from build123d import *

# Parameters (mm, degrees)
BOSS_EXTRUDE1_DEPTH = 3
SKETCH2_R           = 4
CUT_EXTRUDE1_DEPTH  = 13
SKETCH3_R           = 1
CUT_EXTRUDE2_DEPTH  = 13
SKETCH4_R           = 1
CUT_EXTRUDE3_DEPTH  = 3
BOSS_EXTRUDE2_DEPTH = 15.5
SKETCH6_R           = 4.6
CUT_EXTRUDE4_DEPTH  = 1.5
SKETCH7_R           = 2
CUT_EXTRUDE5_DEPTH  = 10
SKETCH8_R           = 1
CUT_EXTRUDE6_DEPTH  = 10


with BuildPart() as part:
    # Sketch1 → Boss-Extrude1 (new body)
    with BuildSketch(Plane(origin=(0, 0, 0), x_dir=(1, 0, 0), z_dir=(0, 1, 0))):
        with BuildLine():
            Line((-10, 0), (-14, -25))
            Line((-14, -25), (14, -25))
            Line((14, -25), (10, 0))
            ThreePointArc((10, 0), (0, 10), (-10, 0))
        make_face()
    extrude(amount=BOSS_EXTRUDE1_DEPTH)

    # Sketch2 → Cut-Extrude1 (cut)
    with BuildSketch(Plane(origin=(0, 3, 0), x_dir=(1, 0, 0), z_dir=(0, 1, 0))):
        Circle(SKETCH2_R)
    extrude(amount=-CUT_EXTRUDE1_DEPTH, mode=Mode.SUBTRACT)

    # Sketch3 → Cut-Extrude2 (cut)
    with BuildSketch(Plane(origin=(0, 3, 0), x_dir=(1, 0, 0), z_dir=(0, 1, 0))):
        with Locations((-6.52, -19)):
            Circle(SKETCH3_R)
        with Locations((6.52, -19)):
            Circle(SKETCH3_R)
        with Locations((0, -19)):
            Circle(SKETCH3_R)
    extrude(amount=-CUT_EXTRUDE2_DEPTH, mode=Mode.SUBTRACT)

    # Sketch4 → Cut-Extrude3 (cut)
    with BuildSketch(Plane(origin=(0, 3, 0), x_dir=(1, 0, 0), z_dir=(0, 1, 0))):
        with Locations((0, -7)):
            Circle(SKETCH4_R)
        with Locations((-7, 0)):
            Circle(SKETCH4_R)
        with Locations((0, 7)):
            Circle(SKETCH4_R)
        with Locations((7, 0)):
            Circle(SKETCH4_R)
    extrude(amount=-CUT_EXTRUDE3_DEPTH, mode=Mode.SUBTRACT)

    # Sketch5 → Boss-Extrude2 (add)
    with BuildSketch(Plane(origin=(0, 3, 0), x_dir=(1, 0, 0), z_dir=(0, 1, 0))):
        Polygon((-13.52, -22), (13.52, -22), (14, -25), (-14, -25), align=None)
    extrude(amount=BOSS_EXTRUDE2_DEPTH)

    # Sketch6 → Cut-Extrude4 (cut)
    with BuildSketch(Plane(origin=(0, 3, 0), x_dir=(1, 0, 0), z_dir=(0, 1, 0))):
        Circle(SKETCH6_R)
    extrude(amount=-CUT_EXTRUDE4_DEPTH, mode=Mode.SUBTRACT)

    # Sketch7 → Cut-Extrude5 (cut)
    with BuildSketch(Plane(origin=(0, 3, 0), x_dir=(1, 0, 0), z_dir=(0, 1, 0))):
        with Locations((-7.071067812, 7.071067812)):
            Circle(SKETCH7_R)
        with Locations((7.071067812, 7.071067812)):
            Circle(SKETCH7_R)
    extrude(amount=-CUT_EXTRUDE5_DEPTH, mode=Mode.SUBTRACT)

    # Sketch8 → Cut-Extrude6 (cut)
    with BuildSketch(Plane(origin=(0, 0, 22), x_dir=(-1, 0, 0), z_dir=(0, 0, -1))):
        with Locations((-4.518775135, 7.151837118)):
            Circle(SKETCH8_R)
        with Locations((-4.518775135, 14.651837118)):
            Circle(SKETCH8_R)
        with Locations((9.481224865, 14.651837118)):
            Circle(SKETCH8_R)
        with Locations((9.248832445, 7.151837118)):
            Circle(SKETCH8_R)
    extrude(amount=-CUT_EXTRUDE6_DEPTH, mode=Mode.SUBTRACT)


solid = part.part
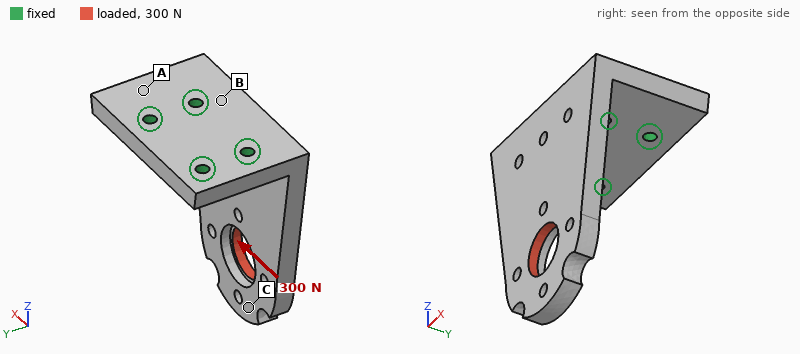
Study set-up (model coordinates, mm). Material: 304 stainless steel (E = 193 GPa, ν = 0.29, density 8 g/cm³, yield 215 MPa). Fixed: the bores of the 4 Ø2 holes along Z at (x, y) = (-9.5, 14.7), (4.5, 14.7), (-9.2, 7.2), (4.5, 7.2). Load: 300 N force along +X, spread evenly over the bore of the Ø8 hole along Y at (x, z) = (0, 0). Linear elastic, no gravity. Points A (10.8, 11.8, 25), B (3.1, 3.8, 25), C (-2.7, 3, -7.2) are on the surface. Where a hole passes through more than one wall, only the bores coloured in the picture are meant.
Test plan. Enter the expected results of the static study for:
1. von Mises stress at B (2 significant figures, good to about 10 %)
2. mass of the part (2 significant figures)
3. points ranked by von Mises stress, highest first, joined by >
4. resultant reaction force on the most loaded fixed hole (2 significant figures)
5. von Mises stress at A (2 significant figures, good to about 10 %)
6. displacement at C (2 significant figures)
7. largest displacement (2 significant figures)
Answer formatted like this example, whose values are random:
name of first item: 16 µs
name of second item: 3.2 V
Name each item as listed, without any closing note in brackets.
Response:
von Mises stress at B: 35 MPa
mass of the part: 26 g
points ranked by von Mises stress, highest first, joined by >: B > A > C
resultant reaction force on the most loaded fixed hole: 500 N
von Mises stress at A: 24 MPa
displacement at C: 23 µm
largest displacement: 25 µm
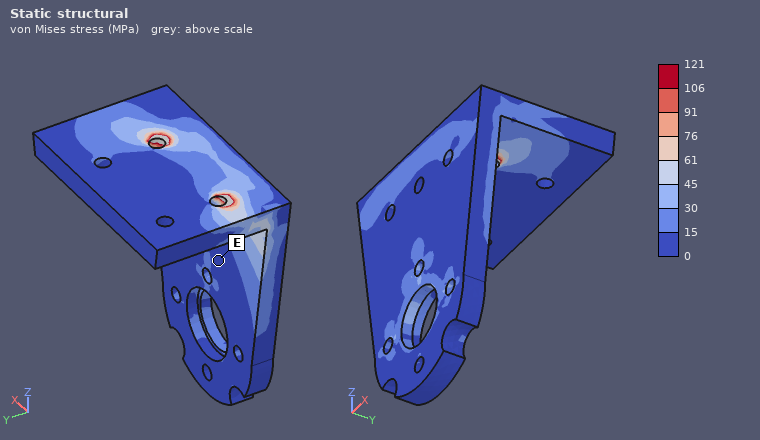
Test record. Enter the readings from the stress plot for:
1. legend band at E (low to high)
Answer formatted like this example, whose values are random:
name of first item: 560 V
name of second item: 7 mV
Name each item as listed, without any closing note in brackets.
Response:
legend band at E: 0 to 15 MPa
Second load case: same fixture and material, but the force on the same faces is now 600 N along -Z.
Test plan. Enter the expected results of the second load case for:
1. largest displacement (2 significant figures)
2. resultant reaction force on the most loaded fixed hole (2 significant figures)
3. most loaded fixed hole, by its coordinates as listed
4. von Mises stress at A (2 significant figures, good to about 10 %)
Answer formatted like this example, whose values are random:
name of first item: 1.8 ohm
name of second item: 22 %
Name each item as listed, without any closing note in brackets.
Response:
largest displacement: 66 µm
resultant reaction force on the most loaded fixed hole: 490 N
most loaded fixed hole, by its coordinates as listed: (4.5, 7.2)
von Mises stress at A: 19 MPa
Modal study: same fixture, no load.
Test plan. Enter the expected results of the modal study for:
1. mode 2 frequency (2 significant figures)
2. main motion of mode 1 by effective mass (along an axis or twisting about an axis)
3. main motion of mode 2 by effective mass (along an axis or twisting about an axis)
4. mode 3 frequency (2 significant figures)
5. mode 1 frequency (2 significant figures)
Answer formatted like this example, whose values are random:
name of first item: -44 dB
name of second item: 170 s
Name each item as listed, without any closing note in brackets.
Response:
mode 2 frequency: 6800 Hz
main motion of mode 1 by effective mass: along Y
main motion of mode 2 by effective mass: along X
mode 3 frequency: 9300 Hz
mode 1 frequency: 2400 Hz
